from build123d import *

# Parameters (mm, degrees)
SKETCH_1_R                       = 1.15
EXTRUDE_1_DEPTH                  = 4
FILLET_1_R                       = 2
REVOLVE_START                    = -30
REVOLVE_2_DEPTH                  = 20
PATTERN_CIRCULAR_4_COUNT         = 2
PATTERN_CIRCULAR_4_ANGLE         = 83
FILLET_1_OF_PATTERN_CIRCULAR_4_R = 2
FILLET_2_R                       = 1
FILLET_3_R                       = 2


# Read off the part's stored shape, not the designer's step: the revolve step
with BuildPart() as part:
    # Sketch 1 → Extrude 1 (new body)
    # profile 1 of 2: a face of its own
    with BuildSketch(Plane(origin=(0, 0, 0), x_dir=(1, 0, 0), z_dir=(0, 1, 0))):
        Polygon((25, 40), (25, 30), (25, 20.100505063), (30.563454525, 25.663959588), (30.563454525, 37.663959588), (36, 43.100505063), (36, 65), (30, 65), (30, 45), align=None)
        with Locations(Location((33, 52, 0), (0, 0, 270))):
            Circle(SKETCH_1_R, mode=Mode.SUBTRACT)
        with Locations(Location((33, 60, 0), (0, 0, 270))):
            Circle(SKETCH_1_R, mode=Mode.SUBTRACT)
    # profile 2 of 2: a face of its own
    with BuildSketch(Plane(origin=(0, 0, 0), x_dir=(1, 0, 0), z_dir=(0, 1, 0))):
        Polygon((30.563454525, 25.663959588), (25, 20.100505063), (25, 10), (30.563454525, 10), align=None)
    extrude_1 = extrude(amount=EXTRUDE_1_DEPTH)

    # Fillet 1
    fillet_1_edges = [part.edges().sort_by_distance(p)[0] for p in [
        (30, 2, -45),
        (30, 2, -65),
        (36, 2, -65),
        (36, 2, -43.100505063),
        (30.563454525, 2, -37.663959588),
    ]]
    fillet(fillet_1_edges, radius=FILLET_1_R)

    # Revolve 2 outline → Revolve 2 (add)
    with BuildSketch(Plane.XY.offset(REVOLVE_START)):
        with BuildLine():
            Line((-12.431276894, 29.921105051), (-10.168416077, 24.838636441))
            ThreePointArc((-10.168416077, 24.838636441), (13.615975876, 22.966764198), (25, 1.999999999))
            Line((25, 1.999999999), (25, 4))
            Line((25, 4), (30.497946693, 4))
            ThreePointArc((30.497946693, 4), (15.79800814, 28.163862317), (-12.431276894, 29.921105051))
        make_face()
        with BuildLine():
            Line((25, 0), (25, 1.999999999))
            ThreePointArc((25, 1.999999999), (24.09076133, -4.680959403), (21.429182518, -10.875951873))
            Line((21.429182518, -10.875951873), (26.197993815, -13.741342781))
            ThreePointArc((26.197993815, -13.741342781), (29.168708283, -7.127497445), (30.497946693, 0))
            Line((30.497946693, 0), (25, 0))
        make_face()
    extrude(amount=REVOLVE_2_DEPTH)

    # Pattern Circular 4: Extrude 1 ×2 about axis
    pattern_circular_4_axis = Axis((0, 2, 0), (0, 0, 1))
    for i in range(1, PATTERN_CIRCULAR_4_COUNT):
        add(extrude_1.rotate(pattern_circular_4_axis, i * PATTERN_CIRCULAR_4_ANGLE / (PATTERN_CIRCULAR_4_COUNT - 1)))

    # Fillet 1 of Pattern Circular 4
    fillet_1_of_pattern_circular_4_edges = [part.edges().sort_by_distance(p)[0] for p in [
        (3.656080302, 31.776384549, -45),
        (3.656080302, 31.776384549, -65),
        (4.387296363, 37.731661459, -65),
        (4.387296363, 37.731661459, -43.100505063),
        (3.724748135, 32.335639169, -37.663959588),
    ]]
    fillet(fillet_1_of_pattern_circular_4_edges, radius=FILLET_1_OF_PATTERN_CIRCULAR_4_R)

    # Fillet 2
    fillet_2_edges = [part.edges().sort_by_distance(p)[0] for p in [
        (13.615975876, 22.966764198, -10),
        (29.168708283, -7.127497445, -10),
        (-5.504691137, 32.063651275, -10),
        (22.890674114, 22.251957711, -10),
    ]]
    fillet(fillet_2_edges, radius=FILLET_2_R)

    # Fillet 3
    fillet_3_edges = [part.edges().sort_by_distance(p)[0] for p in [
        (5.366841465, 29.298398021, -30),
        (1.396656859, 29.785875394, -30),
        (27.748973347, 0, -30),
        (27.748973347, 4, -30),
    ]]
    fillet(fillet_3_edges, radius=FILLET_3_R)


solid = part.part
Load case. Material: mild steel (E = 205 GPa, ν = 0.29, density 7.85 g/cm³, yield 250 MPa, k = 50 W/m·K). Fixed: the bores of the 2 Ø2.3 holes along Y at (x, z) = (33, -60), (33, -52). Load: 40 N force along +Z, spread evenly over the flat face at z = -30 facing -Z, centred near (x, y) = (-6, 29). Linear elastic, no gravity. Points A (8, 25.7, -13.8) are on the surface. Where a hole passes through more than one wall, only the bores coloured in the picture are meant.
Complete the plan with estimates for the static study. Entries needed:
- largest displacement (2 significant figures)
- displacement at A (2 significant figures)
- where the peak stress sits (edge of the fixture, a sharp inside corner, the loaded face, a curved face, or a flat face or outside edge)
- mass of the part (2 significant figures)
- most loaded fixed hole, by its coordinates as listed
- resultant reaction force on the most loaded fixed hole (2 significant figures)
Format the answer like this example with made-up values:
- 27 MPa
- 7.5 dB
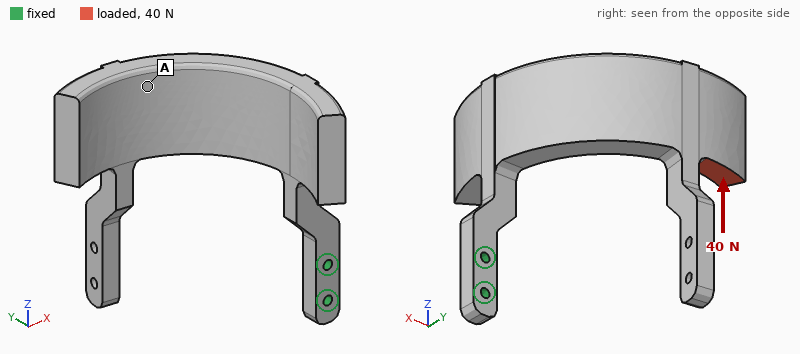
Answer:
- 0.30 mm
- 0.22 mm
- a curved face
- 74 g
- (33, -52)
- 82 N
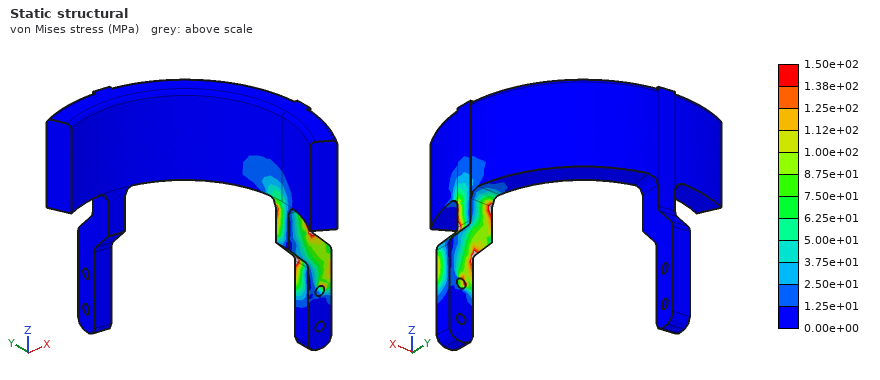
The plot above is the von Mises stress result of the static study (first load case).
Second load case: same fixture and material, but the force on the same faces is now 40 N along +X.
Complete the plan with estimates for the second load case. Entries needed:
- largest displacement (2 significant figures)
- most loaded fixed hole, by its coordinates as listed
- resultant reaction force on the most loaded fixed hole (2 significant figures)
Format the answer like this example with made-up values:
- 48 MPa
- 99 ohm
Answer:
- 0.25 mm
- (33, -52)
- 79 N
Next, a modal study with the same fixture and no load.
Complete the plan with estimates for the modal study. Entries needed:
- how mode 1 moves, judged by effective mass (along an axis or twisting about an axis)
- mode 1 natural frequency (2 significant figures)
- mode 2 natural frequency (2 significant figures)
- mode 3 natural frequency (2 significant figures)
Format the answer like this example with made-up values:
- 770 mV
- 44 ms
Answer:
- along Y
- 290 Hz
- 330 Hz
- 690 Hz
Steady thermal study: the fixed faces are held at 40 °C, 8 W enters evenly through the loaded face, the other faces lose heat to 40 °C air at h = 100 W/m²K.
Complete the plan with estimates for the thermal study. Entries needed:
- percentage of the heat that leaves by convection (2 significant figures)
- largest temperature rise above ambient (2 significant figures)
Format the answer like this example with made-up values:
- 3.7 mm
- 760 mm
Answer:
- 96 %
- 50 K
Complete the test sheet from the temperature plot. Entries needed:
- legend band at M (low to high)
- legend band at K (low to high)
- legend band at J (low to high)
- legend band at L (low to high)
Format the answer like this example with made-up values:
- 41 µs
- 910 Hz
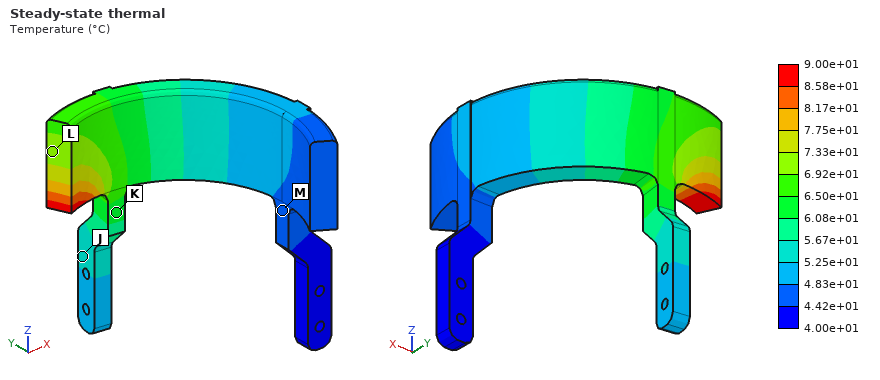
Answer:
- 4.42e+01 to 4.83e+01 °C
- 6.08e+01 to 6.50e+01 °C
- 5.25e+01 to 5.67e+01 °C
- 6.92e+01 to 7.33e+01 °C
